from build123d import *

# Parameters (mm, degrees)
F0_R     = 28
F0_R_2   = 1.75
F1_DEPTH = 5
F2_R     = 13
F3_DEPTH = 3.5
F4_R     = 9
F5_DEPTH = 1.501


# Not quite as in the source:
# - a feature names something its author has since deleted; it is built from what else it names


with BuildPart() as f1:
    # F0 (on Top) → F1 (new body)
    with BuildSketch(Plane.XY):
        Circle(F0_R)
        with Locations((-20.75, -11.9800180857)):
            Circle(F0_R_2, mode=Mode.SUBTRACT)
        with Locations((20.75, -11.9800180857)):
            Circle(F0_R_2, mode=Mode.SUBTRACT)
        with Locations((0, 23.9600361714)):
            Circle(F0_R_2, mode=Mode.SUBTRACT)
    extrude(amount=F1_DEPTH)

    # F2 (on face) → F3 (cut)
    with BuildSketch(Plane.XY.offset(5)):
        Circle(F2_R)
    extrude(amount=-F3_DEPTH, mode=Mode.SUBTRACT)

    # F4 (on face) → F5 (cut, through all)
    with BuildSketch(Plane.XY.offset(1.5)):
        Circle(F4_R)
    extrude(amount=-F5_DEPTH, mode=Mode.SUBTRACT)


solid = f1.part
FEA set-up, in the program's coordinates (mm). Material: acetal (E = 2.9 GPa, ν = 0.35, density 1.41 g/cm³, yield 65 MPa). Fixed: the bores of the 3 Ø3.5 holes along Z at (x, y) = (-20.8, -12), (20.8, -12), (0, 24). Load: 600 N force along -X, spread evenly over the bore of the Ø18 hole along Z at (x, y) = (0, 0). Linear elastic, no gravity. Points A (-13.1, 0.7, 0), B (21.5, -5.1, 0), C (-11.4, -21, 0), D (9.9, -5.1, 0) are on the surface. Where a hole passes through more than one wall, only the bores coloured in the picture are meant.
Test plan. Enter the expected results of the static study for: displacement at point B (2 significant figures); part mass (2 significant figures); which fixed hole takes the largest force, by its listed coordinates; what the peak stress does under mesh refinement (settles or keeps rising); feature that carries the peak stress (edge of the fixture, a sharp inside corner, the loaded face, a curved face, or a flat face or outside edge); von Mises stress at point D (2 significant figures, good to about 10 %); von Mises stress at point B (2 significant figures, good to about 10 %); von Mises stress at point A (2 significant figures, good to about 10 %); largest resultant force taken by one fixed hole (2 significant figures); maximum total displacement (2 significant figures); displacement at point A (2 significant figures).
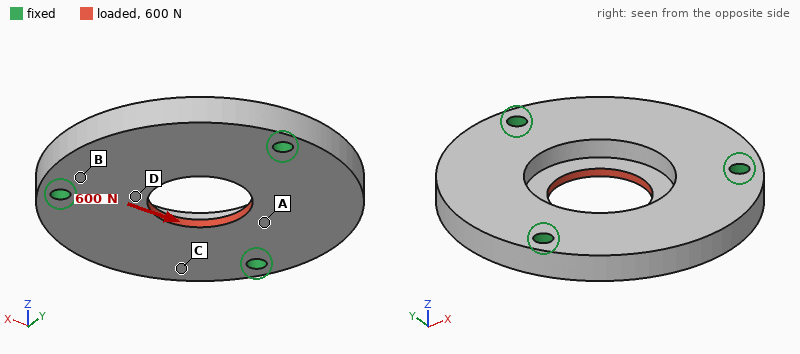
18 µm
14 g
(0, 24)
keeps rising
edge of the fixture
8.1 MPa
3.8 MPa
7.3 MPa
220 N
62 µm
42 µm
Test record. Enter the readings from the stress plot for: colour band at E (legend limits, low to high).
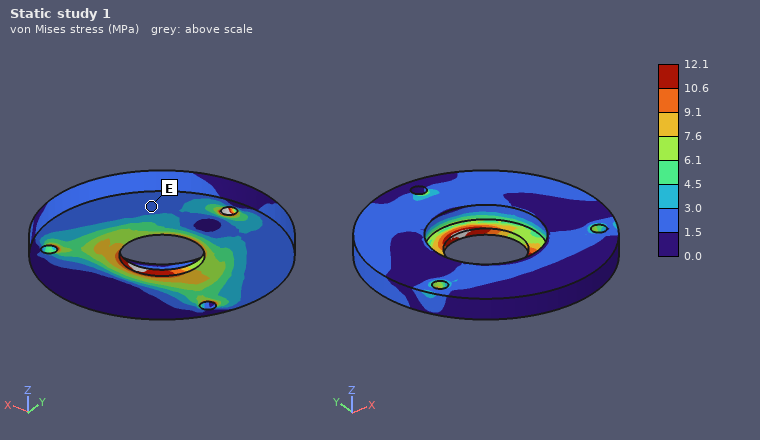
1.5 to 3.0 MPa
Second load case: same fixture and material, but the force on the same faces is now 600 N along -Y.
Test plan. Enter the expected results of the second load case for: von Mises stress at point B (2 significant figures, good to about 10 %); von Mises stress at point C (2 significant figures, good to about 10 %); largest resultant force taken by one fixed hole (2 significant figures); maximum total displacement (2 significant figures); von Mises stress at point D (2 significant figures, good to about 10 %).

2.6 MPa
2.7 MPa
210 N
69 µm
6.2 MPa
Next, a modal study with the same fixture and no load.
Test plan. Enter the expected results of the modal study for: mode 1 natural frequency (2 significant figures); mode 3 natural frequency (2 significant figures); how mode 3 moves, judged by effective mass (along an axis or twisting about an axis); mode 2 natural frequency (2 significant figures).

2700 Hz
3100 Hz
along Z
2700 Hz
